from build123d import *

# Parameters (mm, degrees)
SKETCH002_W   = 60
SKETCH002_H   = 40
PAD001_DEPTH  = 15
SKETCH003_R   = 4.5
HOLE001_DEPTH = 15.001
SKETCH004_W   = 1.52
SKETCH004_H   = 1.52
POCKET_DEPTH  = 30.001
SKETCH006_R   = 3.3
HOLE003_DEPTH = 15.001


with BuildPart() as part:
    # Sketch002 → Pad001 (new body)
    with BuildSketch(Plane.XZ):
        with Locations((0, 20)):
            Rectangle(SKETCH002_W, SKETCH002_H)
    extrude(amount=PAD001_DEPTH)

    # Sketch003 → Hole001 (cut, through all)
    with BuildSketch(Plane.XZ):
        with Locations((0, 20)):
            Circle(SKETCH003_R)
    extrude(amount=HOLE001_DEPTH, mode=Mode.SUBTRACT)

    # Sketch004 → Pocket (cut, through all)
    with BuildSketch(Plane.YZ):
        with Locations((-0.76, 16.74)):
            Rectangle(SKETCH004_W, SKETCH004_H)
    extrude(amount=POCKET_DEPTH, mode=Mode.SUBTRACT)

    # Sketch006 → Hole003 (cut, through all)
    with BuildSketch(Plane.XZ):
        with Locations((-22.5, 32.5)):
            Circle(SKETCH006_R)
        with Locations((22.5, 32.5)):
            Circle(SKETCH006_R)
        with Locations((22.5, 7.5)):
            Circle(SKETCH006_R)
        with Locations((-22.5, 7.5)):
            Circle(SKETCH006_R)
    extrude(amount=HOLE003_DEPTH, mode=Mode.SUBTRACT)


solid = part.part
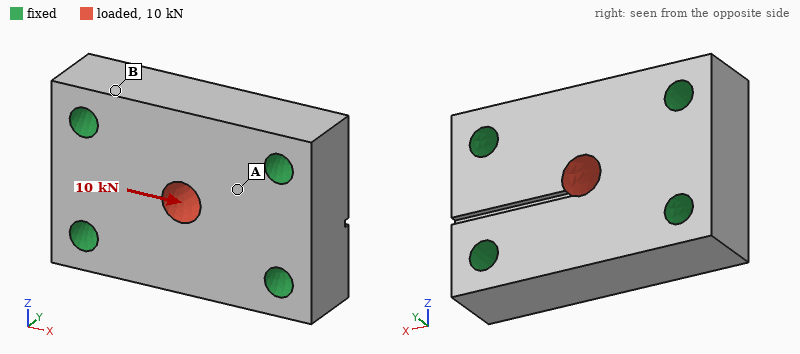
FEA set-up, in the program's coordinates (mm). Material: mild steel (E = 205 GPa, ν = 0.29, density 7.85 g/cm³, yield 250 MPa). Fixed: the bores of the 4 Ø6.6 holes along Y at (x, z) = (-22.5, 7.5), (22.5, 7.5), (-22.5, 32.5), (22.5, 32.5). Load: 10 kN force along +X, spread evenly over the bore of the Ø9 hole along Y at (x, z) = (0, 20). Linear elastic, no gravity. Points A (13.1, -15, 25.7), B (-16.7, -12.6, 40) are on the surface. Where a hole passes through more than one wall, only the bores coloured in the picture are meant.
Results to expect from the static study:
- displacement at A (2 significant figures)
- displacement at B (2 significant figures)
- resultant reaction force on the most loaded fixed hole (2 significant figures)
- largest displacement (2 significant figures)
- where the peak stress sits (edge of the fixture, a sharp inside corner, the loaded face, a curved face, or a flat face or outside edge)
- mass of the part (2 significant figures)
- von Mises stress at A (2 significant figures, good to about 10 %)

0.66 µm
0.30 µm
2.7 kN
1.8 µm
the loaded face
260 g
14 MPa
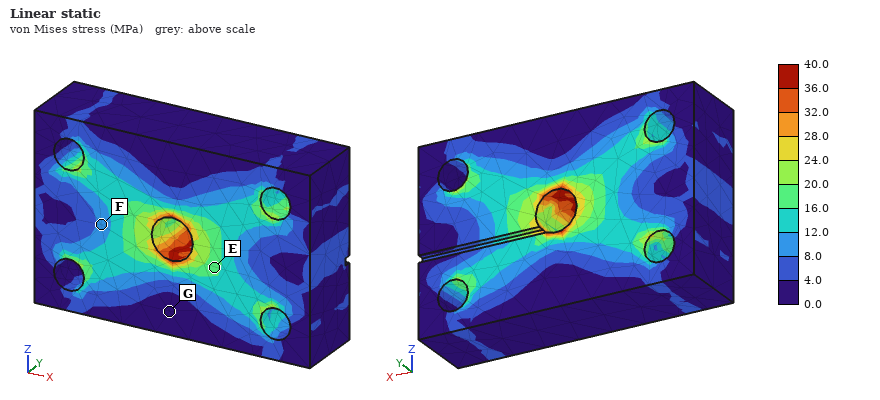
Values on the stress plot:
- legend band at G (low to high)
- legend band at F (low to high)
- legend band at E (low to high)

0.0 to 4.0 MPa
8.0 to 12.0 MPa
16.0 to 20.0 MPa
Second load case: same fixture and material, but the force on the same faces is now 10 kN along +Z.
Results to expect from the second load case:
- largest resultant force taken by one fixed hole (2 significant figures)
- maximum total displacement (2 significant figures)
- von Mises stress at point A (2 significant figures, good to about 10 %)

3.1 kN
3.7 µm
19 MPa
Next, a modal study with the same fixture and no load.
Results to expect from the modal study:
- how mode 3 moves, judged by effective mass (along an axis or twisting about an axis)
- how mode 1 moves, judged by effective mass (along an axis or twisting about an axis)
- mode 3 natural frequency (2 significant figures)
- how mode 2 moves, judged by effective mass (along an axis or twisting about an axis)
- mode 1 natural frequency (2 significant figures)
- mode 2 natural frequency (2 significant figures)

along Z
along Y
34 kHz
twisting about X
26 kHz
31 kHz
